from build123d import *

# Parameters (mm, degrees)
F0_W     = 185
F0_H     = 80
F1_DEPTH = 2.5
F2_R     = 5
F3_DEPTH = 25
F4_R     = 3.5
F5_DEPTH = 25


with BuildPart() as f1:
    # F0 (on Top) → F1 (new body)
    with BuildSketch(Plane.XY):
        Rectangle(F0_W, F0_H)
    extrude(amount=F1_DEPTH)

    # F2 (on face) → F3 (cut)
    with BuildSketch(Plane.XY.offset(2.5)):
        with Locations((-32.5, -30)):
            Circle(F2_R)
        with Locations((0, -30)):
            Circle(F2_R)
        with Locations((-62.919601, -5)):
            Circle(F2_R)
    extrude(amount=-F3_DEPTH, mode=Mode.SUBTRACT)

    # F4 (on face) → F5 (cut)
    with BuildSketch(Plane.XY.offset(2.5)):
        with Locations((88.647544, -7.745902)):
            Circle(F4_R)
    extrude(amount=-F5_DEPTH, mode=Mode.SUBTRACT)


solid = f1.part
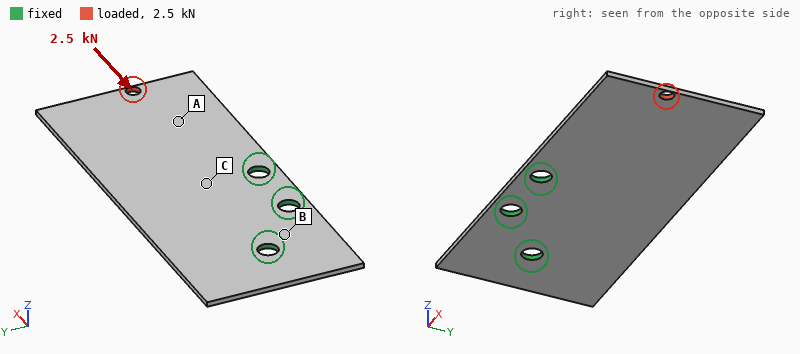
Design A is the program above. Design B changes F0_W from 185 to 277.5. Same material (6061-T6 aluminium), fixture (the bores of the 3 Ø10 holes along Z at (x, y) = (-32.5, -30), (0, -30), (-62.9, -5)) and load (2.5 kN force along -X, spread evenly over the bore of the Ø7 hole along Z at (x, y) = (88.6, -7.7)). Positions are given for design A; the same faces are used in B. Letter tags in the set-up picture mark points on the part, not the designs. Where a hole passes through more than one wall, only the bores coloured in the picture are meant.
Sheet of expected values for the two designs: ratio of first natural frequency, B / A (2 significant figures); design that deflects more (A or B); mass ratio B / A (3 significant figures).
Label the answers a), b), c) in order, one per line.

a) 0.48
b) A
c) 1.51
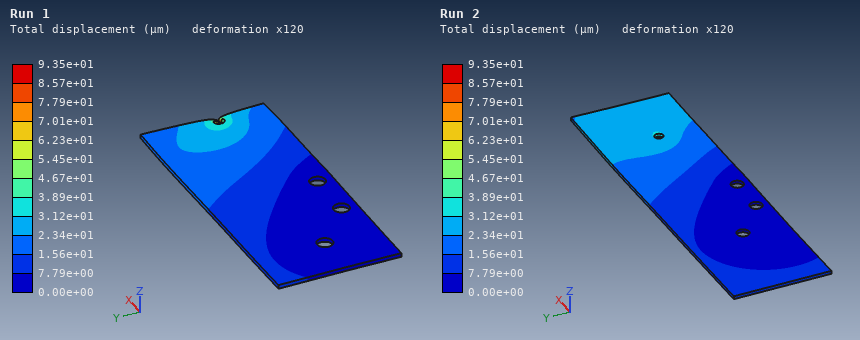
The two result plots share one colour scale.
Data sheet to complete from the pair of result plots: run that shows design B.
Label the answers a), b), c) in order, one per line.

a) Run 2
